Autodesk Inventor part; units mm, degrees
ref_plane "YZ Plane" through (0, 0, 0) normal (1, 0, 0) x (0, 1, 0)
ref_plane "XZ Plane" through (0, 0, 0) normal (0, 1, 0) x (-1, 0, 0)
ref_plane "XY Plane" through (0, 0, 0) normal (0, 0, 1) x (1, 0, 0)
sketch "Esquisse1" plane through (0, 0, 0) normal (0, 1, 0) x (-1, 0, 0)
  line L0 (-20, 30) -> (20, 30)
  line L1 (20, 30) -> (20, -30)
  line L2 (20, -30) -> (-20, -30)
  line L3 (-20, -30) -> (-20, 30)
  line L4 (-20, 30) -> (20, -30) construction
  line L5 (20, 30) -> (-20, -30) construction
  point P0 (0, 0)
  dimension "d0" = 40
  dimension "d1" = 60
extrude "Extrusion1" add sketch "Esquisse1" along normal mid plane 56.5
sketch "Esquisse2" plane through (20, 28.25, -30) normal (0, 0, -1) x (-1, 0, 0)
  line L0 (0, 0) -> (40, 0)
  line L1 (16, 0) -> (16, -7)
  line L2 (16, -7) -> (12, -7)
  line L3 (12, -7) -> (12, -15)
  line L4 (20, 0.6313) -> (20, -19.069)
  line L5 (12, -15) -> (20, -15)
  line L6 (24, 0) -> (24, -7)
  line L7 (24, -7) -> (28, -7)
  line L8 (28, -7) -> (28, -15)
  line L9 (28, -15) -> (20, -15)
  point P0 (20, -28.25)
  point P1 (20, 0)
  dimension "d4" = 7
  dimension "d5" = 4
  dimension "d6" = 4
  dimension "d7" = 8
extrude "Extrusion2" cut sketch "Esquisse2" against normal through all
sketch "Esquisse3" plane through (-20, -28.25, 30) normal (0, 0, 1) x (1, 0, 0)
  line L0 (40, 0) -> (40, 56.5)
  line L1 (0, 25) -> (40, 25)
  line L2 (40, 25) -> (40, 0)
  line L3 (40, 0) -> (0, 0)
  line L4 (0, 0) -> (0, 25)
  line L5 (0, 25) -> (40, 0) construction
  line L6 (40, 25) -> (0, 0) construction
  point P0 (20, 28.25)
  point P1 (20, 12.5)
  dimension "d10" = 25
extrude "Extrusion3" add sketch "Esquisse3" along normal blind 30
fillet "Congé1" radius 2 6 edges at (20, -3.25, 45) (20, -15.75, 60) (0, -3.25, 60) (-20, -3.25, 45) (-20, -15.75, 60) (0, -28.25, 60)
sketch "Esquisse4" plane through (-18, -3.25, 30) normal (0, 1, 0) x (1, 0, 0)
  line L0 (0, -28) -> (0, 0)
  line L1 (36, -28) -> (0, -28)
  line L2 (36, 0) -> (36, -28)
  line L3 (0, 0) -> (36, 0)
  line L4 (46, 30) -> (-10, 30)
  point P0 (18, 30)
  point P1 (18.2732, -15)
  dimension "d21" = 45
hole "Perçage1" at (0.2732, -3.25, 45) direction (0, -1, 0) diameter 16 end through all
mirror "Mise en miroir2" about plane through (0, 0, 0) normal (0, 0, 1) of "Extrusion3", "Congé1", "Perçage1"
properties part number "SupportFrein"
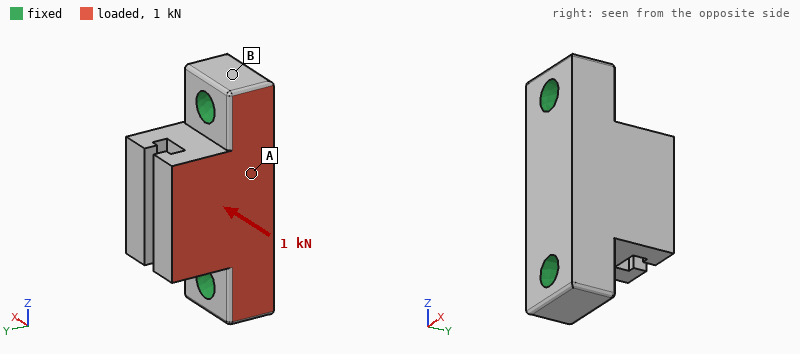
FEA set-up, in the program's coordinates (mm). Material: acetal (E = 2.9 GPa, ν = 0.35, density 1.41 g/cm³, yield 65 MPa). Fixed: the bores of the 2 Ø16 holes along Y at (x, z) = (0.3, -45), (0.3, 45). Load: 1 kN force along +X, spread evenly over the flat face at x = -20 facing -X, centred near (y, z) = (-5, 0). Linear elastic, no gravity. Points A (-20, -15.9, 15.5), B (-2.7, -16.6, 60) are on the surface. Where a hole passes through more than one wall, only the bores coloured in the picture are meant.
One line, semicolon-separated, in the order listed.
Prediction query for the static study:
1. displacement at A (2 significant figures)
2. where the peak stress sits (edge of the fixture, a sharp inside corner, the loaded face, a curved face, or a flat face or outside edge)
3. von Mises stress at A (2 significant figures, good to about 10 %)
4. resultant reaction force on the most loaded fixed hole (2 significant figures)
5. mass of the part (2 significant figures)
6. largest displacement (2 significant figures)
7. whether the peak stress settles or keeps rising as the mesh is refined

19 µm; edge of the fixture; 0.75 MPa; 500 N; 250 g; 68 µm; keeps rising
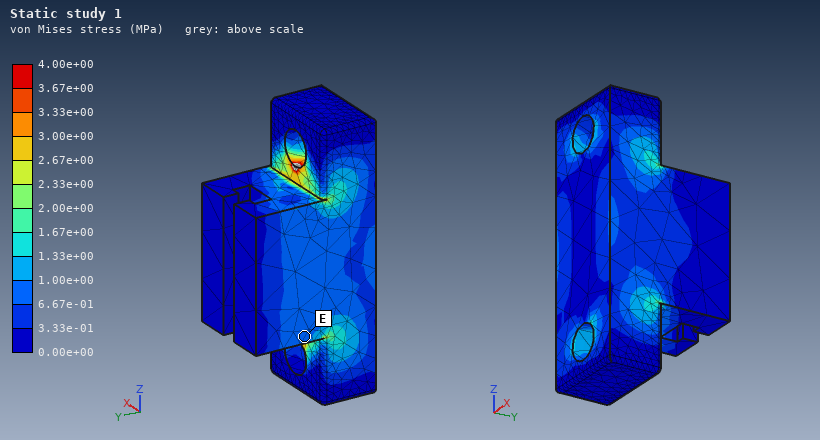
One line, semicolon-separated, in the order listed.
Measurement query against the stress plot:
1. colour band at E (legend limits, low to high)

6.67e-01 to 1.00e+00 MPa
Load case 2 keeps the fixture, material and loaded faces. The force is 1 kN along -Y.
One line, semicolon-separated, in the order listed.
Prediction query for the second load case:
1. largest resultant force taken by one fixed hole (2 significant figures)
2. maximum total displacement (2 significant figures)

510 N; 74 µm
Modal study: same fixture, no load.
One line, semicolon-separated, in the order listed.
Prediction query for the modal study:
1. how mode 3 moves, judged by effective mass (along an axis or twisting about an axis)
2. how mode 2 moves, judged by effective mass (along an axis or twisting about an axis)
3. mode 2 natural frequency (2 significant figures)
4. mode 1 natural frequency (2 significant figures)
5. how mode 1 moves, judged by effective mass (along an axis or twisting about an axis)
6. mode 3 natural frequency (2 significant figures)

along Z; along Y; 3200 Hz; 1700 Hz; along X; 3700 Hz
